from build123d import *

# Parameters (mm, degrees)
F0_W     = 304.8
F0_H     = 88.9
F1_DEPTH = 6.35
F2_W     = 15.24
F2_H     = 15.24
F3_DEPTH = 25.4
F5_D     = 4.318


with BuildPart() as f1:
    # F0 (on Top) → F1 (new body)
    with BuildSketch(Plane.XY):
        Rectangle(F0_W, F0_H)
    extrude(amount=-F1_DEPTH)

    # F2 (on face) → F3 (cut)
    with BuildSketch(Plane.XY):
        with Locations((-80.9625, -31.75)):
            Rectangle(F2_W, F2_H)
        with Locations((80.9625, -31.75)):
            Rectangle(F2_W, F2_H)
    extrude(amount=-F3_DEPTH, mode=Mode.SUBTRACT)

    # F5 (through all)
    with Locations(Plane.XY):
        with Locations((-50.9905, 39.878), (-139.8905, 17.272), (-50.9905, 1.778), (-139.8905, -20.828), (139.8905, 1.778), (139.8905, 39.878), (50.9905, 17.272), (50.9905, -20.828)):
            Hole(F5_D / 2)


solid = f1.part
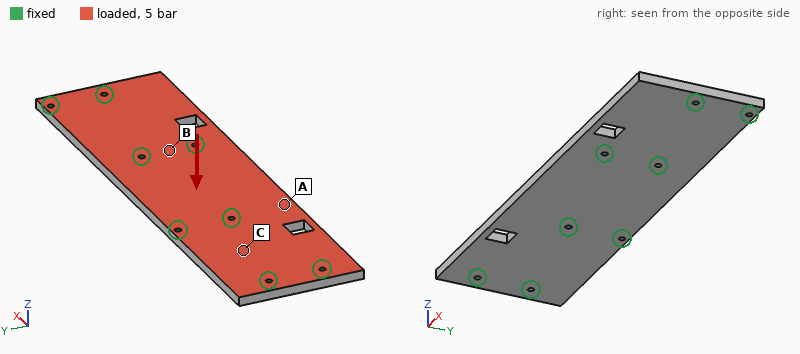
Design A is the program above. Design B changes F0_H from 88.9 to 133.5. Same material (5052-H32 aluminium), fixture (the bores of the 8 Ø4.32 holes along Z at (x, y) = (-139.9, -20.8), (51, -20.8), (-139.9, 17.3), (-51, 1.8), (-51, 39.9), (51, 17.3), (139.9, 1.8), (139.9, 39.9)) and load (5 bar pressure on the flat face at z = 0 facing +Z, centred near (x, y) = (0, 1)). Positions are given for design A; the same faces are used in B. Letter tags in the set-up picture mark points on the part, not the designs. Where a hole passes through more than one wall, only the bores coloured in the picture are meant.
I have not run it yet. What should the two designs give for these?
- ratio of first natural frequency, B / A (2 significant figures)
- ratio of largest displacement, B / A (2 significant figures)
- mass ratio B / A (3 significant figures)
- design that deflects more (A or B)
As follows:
0.58
3.3
1.51
B
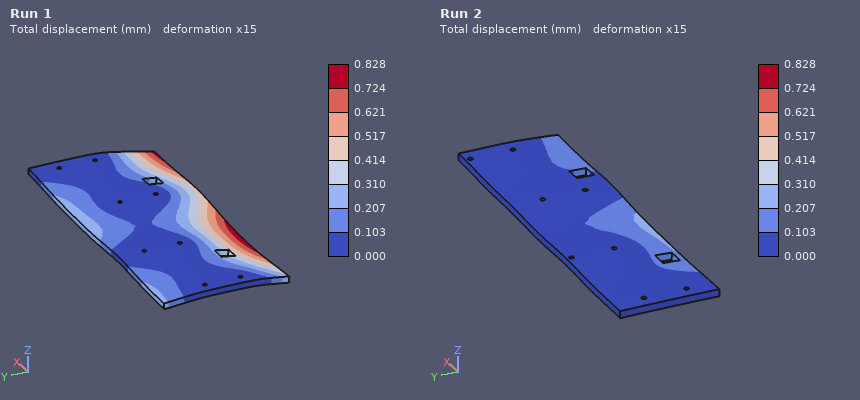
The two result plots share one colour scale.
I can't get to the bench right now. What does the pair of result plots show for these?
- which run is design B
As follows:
Run 1
